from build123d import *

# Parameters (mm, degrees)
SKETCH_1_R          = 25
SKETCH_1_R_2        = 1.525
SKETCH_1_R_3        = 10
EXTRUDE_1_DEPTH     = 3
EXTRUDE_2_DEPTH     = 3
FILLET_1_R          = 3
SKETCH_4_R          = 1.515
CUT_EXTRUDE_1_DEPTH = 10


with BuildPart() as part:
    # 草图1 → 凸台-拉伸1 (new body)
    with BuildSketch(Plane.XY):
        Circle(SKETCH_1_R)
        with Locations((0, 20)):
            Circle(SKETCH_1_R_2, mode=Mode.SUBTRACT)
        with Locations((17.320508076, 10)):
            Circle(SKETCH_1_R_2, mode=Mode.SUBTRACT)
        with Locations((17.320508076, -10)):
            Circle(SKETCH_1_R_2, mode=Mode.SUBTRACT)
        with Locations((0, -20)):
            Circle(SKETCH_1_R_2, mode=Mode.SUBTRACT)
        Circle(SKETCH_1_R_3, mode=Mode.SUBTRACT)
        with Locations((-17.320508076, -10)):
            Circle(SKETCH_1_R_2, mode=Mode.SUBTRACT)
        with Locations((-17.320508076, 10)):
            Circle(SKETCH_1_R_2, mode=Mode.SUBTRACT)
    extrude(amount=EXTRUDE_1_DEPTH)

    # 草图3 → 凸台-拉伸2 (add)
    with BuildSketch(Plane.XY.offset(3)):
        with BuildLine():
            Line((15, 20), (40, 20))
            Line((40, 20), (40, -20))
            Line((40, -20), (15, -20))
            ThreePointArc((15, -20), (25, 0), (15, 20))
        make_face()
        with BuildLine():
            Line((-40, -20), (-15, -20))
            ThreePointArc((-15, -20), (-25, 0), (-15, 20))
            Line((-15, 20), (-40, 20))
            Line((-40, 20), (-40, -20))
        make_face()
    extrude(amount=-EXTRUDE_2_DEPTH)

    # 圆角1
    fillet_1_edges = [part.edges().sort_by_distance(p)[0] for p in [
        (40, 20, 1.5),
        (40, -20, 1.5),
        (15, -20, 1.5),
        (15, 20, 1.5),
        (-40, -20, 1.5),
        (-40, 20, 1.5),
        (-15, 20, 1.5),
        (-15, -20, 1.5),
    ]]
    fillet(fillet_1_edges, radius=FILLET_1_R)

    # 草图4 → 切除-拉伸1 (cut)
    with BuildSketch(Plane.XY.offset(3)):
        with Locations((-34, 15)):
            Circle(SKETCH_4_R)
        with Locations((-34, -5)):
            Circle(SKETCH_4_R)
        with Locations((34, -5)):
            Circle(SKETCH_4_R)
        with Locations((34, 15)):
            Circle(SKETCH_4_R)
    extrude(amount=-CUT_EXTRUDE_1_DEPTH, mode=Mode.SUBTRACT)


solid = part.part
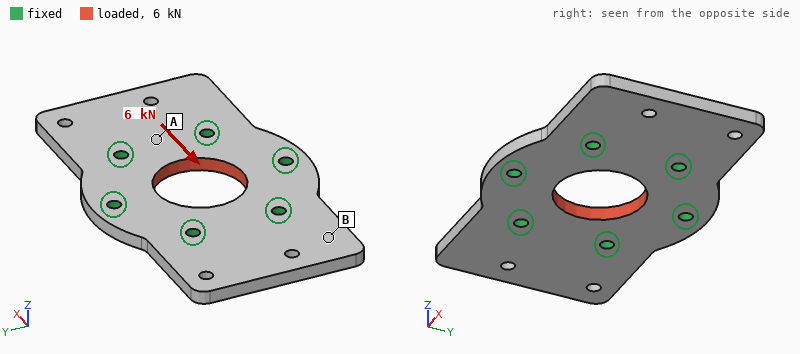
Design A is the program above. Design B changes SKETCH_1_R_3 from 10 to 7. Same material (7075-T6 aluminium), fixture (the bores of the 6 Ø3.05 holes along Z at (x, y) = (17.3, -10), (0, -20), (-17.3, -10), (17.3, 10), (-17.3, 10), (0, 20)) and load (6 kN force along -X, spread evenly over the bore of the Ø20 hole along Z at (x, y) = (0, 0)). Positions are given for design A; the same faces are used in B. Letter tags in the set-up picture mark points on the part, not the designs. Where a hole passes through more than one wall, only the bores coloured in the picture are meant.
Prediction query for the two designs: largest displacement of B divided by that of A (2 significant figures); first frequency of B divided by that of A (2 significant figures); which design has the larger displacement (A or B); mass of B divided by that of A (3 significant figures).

1.3
1.0
B
1.05
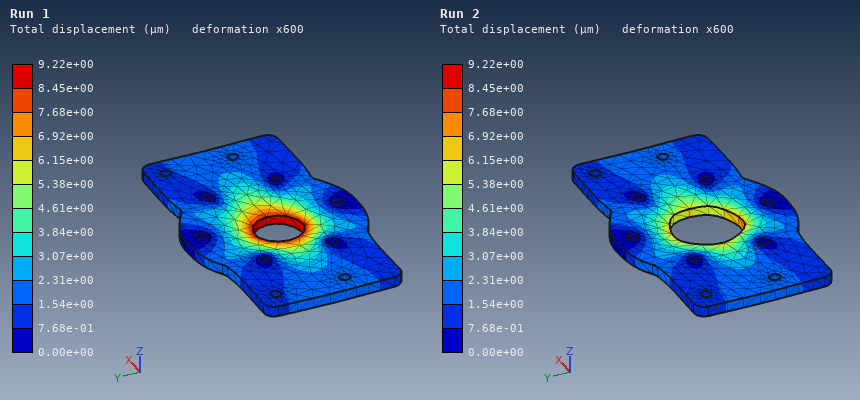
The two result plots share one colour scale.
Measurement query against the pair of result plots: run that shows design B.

Run 1
